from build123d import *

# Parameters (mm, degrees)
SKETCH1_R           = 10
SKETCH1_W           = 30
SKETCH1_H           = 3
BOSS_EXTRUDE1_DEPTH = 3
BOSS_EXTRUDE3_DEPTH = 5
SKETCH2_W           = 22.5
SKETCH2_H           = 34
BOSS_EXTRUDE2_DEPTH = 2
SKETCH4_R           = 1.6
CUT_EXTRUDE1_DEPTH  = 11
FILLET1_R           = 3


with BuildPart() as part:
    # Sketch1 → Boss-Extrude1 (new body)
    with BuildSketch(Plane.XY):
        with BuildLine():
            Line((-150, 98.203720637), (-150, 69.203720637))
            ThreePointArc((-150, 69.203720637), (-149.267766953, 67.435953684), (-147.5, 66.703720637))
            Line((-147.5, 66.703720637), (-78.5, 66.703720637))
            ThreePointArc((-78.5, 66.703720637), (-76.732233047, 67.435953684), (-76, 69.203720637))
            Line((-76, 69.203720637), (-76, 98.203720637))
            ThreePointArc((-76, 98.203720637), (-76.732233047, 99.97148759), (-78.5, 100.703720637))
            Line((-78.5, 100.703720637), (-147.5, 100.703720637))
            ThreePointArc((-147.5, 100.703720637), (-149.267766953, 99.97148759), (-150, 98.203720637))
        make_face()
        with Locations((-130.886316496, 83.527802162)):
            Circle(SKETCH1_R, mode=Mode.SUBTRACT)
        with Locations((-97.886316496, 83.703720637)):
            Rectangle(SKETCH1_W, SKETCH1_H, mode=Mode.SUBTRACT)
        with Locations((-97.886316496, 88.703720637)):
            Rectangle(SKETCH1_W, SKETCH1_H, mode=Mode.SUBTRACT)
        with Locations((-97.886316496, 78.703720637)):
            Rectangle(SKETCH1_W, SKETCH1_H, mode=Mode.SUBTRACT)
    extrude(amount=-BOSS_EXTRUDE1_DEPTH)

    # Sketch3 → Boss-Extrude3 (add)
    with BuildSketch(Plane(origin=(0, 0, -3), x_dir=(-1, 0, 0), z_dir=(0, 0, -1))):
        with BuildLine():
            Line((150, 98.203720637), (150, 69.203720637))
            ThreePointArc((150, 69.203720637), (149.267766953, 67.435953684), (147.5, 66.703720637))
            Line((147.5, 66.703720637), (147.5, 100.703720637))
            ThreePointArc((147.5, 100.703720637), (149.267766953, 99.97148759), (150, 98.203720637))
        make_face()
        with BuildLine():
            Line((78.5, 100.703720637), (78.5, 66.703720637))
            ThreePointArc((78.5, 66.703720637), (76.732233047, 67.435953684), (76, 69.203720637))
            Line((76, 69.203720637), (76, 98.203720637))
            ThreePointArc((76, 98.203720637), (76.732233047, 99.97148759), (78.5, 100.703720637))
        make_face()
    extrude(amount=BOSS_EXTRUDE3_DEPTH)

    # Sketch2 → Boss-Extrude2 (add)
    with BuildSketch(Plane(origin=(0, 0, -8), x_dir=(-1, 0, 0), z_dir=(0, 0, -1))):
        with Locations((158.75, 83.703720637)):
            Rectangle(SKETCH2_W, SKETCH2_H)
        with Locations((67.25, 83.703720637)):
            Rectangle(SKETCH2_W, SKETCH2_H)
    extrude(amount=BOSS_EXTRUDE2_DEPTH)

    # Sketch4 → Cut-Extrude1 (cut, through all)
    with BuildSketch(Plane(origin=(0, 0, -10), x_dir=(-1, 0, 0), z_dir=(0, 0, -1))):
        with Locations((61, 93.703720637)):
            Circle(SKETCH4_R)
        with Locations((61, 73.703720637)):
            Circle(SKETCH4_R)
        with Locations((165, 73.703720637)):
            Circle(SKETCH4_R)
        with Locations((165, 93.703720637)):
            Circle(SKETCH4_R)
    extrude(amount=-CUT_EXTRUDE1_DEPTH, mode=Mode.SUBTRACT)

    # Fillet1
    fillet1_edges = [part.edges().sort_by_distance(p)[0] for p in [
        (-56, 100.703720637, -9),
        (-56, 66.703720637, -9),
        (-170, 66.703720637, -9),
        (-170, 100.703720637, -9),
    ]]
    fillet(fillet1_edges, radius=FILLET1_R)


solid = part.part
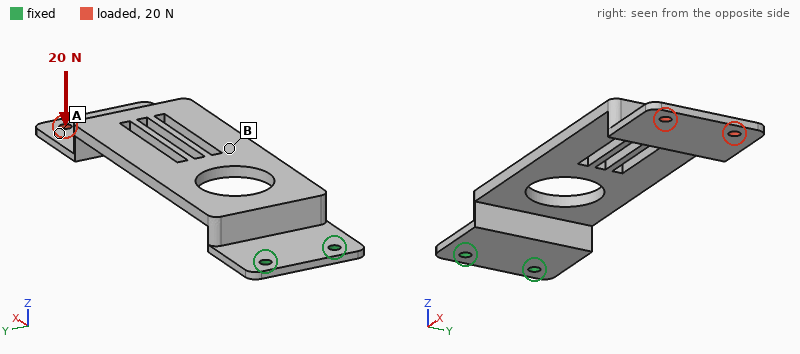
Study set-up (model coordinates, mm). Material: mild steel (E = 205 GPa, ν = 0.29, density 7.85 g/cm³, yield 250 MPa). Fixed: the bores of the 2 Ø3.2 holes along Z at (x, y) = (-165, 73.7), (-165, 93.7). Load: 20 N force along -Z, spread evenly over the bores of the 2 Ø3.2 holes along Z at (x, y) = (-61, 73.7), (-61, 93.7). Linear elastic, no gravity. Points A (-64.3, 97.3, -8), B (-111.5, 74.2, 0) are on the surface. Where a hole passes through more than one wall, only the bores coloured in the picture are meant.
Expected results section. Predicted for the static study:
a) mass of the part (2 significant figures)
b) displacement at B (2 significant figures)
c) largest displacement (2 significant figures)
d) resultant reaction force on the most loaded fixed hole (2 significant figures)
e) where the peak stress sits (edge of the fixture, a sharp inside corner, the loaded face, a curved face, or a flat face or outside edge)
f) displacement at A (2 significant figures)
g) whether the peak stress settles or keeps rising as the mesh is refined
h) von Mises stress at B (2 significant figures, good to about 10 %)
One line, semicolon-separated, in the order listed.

75 g; 0.44 mm; 1.3 mm; 15 N; edge of the fixture; 1.1 mm; keeps rising; 26 MPa
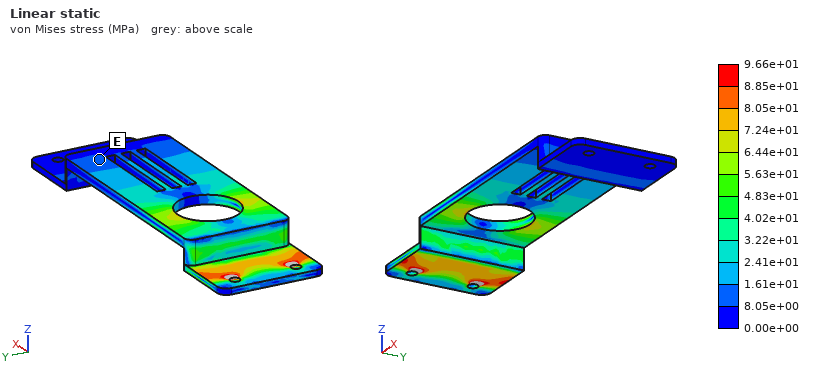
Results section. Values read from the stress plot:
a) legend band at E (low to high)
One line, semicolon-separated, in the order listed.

8.05e+00 to 1.61e+01 MPa
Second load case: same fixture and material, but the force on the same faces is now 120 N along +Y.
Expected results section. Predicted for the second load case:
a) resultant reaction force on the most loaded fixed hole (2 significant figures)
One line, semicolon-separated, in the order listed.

580 N
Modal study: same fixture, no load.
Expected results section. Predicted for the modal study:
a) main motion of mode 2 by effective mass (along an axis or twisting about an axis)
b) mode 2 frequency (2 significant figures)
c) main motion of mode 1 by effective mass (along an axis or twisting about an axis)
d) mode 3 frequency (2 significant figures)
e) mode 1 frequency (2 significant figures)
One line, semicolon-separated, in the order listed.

along Y; 700 Hz; along Z; 1000 Hz; 140 Hz
